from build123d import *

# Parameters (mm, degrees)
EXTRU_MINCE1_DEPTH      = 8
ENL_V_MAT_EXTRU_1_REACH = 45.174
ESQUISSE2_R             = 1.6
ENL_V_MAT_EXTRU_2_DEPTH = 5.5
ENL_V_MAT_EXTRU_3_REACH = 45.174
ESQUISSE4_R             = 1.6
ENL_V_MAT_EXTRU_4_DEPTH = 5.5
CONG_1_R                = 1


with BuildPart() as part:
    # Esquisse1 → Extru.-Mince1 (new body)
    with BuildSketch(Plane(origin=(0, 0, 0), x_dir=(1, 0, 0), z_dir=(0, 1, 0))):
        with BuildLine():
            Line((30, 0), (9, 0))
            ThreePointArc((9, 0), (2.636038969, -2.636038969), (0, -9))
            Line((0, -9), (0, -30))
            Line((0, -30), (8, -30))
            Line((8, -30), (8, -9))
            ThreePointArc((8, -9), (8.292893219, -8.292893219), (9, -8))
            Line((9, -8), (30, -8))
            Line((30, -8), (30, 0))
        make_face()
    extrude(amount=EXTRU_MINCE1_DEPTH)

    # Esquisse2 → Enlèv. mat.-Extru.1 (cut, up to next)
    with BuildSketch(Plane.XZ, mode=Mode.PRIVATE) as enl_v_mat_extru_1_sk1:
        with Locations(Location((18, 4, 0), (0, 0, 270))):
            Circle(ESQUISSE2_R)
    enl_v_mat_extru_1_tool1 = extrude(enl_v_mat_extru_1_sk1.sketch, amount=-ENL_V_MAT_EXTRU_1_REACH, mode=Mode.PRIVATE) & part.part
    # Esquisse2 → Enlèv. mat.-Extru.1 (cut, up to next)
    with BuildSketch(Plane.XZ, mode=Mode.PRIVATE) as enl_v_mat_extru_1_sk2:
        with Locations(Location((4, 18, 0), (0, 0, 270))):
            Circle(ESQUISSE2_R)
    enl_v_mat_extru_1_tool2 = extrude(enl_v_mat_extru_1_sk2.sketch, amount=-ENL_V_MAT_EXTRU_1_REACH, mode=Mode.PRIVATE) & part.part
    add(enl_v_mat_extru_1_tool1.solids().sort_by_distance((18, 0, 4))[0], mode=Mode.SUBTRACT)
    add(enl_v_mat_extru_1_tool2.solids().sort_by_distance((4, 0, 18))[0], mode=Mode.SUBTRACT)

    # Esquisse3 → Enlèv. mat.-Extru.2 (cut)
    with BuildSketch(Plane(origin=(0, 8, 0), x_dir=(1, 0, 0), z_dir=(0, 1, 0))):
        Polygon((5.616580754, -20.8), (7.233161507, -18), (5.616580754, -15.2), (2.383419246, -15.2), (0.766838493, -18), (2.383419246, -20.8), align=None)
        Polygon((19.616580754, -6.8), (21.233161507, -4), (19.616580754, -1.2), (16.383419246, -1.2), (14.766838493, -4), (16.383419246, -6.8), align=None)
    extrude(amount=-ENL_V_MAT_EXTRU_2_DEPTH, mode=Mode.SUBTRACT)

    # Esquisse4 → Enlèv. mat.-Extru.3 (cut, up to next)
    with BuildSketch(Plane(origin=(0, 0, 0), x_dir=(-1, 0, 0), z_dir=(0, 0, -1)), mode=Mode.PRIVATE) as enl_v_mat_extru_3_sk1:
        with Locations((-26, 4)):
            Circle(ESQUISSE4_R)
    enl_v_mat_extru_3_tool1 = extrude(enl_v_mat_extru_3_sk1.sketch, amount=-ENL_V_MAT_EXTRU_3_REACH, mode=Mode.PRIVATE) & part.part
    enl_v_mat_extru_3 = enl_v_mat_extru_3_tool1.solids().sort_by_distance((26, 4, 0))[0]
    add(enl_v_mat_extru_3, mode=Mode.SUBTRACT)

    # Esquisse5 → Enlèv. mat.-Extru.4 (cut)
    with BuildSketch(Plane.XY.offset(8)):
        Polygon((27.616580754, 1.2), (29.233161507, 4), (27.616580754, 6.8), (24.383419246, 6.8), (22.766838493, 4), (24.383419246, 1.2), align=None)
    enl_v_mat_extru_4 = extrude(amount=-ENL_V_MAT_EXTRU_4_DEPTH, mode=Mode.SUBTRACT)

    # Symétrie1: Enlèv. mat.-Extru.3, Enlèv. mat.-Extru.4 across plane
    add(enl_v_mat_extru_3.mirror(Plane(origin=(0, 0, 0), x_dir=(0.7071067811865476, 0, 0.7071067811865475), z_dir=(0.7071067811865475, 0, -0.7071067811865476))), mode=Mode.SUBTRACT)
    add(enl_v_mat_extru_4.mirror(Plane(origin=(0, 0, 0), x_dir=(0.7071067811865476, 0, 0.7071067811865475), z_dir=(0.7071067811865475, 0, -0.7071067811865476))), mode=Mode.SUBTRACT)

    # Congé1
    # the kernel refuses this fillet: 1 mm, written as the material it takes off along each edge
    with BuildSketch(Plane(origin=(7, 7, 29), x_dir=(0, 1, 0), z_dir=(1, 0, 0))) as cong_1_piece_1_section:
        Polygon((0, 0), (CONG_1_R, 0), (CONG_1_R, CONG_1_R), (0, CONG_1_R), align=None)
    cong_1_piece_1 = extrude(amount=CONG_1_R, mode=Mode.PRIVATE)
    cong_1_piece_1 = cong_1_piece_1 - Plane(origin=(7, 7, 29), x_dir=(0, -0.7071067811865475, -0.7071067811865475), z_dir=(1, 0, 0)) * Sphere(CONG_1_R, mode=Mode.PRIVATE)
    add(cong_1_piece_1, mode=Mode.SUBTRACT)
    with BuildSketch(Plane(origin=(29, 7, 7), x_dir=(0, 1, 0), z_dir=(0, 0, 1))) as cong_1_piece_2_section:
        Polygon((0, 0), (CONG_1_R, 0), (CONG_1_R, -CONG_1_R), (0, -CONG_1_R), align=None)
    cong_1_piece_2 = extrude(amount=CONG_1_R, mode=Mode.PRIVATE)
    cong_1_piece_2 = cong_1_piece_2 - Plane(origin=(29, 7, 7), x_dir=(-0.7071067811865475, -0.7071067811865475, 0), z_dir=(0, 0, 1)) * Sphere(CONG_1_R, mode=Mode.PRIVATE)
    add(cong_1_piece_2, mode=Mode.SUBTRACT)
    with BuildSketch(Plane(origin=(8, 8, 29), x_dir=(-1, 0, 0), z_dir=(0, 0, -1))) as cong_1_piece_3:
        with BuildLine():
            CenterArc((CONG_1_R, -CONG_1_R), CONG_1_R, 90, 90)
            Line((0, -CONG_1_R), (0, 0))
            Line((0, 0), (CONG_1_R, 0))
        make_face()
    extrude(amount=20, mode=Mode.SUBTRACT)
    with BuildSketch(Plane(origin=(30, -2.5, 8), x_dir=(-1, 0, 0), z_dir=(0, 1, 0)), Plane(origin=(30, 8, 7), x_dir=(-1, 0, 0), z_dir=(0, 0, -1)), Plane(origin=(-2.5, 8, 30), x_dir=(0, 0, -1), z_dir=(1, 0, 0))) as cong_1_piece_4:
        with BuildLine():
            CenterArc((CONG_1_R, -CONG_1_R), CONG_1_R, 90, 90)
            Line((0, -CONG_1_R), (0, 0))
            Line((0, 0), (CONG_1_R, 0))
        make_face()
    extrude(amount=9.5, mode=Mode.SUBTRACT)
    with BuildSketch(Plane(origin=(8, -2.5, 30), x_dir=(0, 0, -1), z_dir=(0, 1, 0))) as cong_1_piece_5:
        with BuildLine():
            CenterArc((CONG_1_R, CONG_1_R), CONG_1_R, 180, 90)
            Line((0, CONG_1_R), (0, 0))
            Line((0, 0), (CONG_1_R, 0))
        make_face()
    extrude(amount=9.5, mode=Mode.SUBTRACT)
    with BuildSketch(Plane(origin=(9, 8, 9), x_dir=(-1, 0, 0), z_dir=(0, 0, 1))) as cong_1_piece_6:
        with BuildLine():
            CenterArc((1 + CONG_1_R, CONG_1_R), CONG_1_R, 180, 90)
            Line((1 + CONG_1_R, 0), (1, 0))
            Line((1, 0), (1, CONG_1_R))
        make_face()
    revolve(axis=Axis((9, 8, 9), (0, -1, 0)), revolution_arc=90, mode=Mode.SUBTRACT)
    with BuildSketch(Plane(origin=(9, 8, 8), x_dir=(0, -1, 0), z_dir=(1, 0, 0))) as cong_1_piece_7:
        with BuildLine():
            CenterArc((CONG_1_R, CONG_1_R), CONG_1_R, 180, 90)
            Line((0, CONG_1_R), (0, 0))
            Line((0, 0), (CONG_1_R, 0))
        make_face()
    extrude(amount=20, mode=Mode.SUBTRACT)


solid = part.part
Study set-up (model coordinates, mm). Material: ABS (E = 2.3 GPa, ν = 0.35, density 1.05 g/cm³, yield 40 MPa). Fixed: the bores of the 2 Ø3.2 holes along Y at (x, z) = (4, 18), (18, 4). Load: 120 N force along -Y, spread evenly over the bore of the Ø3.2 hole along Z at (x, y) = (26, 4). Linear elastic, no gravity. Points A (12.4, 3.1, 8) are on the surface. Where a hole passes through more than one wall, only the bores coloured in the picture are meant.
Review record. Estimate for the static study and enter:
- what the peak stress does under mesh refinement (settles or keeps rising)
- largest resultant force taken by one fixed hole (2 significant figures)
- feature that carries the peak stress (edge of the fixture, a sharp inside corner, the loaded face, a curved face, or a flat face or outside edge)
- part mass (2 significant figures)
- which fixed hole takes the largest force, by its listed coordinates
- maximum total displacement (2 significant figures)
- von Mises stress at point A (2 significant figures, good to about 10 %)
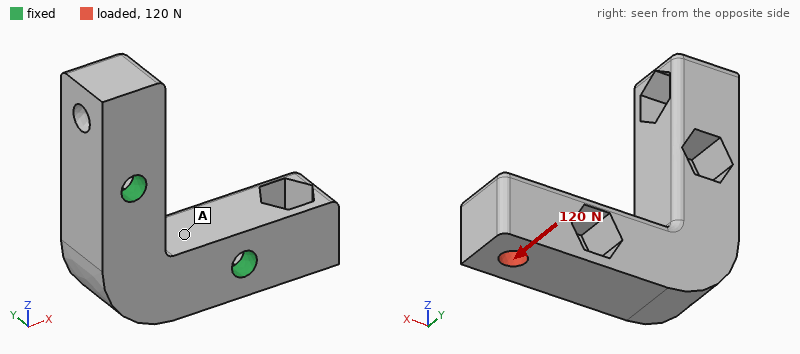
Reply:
keeps rising
150 N
edge of the fixture
2.6 g
(18, 4)
0.31 mm
4.1 MPa
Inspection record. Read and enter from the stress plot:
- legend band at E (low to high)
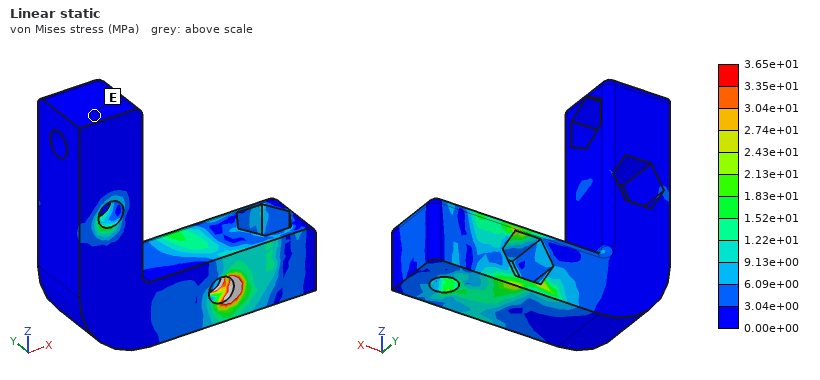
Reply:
0.00e+00 to 3.04e+00 MPa
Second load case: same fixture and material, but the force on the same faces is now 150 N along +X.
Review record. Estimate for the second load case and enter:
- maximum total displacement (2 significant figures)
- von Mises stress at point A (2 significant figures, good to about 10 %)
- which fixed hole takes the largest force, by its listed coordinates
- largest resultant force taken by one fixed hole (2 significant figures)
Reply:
0.14 mm
1.3 MPa
(18, 4)
140 N
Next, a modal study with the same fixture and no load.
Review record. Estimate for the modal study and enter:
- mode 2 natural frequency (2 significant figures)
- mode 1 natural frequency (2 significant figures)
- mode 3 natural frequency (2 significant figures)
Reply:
6200 Hz
3900 Hz
6800 Hz
